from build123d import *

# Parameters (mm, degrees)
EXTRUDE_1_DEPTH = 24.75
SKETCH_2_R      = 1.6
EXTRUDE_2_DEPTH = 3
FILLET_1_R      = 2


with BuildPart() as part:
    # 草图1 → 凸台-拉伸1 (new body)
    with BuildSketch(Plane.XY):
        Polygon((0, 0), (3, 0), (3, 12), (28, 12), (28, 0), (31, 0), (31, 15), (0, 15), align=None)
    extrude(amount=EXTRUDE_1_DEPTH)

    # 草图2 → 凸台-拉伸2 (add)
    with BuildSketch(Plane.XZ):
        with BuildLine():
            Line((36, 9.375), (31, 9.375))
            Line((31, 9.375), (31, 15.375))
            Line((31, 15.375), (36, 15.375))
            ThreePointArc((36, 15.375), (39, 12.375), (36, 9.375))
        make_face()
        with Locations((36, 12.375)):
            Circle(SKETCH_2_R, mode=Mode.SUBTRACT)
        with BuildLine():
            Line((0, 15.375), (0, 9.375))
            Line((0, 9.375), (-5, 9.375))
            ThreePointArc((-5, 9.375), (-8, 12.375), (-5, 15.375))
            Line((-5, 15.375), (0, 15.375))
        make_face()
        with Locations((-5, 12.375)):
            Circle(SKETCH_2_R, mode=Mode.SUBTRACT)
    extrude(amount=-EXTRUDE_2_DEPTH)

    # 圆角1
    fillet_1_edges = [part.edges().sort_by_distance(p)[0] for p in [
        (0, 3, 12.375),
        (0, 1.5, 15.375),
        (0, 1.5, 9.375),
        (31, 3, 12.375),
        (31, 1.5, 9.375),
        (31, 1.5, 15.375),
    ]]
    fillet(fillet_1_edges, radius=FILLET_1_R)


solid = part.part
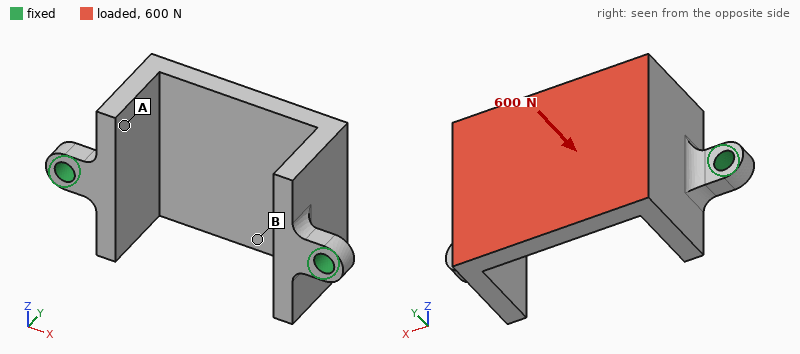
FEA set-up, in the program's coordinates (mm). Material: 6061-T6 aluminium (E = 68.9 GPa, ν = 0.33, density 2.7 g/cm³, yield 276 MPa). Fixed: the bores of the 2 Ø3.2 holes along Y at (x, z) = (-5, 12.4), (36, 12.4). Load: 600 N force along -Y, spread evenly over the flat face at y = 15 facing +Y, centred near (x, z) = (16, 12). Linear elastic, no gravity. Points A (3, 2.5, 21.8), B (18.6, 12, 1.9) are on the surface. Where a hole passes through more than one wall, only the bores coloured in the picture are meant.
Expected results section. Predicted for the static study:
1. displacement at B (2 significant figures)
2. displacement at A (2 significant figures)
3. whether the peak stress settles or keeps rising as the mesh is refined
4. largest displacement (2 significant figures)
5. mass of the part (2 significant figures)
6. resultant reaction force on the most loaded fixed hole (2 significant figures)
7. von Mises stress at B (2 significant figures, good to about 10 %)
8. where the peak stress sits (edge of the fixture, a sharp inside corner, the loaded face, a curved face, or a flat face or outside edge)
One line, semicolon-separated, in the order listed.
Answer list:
19 µm; 7.1 µm; keeps rising; 20 µm; 12 g; 350 N; 16 MPa; edge of the fixture
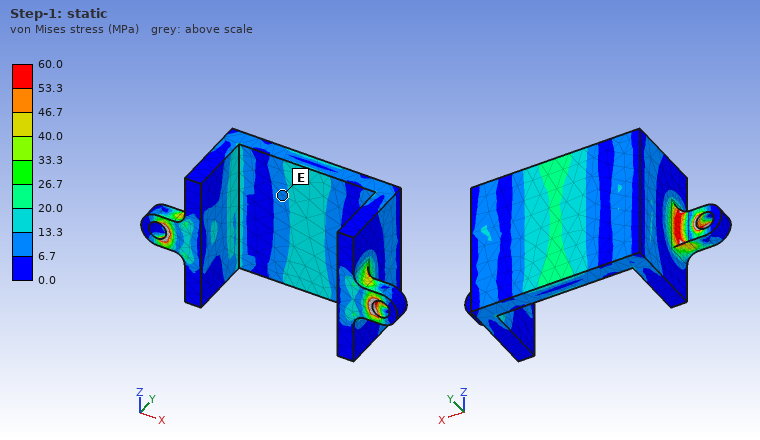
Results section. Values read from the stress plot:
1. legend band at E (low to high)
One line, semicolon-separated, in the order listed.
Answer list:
6.7 to 13.3 MPa
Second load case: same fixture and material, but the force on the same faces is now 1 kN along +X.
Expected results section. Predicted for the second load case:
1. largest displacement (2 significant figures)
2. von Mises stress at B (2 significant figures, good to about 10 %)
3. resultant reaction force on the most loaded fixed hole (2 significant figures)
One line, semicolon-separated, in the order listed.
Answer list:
71 µm; 23 MPa; 590 N
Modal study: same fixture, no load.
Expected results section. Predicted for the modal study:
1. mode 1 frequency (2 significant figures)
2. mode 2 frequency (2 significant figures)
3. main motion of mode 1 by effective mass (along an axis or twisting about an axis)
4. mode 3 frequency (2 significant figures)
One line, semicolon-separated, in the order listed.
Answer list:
3000 Hz; 6800 Hz; along Z; 7000 Hz
